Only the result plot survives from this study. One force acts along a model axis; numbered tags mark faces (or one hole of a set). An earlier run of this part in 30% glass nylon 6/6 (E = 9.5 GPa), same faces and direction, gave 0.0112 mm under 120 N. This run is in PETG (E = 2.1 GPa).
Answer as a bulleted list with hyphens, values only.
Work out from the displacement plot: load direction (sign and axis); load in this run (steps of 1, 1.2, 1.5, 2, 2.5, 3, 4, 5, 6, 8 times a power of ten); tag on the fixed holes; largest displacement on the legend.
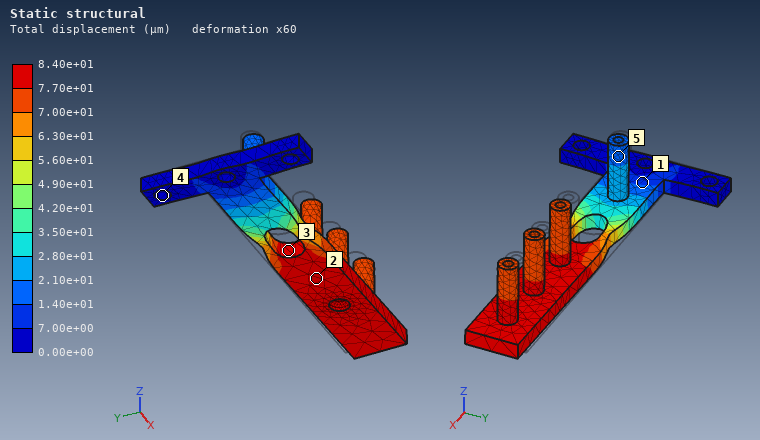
- +X
- 200 N
- 4
- 8.40e+01 µm
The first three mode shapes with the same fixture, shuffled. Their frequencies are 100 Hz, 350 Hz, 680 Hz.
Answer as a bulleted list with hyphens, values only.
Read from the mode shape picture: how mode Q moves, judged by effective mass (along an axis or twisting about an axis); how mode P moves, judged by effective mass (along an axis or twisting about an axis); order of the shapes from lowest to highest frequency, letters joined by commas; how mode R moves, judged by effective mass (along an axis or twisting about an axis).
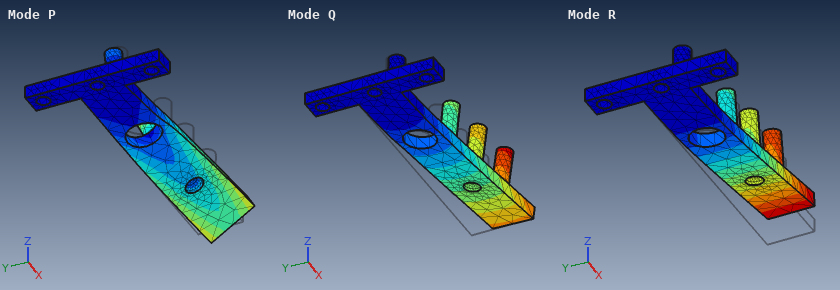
- along Y
- twisting about X
- R, Q, P
- along Z
